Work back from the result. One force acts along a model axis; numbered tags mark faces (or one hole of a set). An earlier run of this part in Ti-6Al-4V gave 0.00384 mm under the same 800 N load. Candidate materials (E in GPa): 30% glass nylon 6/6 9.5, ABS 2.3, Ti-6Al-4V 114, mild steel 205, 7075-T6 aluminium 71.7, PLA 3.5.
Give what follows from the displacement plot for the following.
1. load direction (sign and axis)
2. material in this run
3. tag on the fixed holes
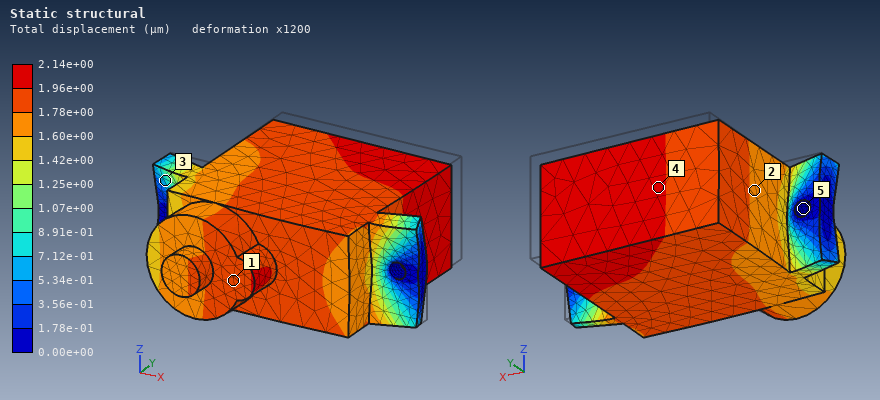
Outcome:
-Y
mild steel
5
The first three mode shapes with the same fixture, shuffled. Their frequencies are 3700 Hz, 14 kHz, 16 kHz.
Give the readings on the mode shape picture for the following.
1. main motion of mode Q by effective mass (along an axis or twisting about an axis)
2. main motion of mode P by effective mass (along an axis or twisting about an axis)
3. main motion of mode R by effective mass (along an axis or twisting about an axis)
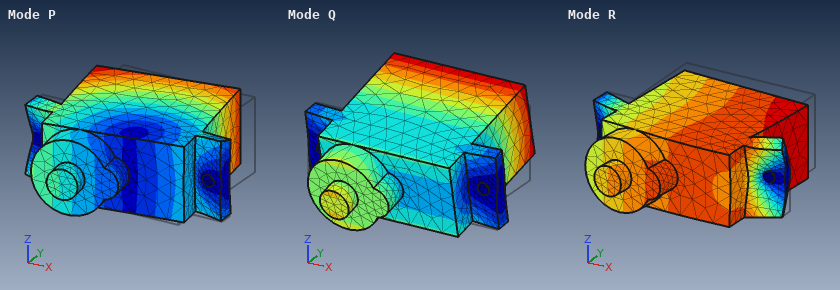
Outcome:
along Z
along X
along Y
